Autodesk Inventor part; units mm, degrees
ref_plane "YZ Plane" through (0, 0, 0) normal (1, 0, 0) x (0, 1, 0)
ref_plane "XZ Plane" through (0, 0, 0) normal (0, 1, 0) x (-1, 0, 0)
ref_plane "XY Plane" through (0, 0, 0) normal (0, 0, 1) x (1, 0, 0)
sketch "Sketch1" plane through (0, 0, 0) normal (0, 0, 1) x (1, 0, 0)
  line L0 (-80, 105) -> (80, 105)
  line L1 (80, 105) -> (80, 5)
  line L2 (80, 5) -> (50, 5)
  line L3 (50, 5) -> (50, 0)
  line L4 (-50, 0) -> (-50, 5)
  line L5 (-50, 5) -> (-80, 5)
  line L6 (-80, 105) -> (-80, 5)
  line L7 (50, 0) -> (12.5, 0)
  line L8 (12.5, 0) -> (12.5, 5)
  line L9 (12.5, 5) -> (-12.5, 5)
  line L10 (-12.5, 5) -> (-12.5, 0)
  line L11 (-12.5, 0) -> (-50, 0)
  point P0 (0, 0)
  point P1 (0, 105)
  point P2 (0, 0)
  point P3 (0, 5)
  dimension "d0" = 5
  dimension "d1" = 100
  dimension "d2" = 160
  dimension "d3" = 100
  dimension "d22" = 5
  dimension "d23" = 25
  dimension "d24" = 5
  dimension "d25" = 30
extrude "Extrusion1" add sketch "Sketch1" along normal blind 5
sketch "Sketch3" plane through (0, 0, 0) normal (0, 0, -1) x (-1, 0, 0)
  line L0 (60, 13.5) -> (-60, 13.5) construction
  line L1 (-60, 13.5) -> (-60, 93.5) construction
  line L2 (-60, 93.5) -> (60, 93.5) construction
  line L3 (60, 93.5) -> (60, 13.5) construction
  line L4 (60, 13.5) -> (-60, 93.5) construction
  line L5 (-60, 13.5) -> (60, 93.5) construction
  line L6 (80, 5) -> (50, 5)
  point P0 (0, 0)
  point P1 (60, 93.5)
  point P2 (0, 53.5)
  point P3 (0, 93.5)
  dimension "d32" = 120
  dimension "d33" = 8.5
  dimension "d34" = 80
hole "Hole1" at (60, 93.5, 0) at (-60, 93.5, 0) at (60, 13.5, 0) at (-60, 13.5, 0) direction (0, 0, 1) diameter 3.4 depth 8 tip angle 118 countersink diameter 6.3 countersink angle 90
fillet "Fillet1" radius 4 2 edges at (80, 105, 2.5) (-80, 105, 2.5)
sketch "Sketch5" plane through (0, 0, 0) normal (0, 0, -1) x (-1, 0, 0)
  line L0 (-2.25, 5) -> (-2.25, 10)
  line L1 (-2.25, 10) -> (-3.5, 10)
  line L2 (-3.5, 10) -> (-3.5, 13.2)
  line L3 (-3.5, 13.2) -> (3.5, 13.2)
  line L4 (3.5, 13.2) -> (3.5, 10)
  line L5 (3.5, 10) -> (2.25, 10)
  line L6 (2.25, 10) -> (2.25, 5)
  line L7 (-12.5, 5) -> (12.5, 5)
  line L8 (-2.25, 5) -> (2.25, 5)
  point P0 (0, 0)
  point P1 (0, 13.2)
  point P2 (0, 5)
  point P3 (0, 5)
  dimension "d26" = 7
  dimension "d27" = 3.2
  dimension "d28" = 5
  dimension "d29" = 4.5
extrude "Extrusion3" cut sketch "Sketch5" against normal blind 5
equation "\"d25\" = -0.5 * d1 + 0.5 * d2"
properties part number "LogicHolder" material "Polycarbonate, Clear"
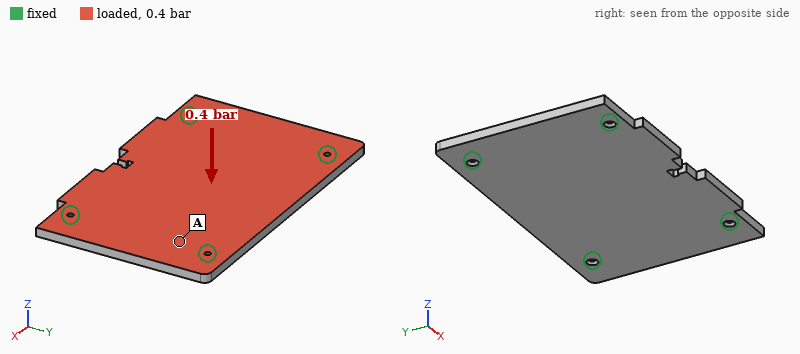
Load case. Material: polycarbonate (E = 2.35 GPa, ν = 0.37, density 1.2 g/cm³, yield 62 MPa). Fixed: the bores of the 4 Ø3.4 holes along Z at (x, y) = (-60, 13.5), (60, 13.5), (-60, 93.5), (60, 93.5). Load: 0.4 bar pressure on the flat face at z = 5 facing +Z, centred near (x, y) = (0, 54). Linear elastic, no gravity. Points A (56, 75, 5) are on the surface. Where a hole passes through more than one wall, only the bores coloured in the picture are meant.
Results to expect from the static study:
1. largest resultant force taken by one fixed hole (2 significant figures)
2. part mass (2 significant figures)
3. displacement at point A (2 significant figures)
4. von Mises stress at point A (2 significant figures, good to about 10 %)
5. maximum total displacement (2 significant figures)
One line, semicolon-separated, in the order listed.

180 N; 98 g; 0.36 mm; 4.2 MPa; 1.7 mm
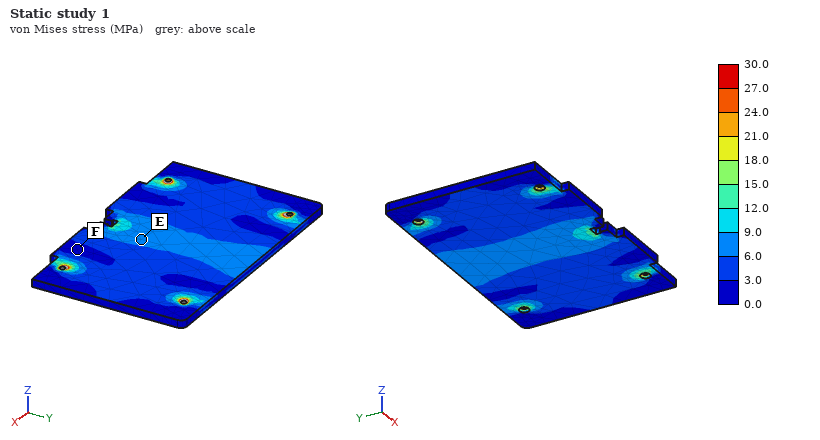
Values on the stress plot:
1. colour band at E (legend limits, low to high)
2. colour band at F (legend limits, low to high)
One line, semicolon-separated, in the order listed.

6.0 to 9.0 MPa; 0.0 to 3.0 MPa
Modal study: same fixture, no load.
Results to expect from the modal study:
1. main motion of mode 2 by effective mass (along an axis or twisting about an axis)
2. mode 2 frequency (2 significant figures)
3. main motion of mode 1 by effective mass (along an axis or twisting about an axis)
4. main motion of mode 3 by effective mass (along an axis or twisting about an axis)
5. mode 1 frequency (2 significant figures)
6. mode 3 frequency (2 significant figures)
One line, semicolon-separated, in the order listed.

twisting about X; 560 Hz; along Z; along Z; 360 Hz; 800 Hz
